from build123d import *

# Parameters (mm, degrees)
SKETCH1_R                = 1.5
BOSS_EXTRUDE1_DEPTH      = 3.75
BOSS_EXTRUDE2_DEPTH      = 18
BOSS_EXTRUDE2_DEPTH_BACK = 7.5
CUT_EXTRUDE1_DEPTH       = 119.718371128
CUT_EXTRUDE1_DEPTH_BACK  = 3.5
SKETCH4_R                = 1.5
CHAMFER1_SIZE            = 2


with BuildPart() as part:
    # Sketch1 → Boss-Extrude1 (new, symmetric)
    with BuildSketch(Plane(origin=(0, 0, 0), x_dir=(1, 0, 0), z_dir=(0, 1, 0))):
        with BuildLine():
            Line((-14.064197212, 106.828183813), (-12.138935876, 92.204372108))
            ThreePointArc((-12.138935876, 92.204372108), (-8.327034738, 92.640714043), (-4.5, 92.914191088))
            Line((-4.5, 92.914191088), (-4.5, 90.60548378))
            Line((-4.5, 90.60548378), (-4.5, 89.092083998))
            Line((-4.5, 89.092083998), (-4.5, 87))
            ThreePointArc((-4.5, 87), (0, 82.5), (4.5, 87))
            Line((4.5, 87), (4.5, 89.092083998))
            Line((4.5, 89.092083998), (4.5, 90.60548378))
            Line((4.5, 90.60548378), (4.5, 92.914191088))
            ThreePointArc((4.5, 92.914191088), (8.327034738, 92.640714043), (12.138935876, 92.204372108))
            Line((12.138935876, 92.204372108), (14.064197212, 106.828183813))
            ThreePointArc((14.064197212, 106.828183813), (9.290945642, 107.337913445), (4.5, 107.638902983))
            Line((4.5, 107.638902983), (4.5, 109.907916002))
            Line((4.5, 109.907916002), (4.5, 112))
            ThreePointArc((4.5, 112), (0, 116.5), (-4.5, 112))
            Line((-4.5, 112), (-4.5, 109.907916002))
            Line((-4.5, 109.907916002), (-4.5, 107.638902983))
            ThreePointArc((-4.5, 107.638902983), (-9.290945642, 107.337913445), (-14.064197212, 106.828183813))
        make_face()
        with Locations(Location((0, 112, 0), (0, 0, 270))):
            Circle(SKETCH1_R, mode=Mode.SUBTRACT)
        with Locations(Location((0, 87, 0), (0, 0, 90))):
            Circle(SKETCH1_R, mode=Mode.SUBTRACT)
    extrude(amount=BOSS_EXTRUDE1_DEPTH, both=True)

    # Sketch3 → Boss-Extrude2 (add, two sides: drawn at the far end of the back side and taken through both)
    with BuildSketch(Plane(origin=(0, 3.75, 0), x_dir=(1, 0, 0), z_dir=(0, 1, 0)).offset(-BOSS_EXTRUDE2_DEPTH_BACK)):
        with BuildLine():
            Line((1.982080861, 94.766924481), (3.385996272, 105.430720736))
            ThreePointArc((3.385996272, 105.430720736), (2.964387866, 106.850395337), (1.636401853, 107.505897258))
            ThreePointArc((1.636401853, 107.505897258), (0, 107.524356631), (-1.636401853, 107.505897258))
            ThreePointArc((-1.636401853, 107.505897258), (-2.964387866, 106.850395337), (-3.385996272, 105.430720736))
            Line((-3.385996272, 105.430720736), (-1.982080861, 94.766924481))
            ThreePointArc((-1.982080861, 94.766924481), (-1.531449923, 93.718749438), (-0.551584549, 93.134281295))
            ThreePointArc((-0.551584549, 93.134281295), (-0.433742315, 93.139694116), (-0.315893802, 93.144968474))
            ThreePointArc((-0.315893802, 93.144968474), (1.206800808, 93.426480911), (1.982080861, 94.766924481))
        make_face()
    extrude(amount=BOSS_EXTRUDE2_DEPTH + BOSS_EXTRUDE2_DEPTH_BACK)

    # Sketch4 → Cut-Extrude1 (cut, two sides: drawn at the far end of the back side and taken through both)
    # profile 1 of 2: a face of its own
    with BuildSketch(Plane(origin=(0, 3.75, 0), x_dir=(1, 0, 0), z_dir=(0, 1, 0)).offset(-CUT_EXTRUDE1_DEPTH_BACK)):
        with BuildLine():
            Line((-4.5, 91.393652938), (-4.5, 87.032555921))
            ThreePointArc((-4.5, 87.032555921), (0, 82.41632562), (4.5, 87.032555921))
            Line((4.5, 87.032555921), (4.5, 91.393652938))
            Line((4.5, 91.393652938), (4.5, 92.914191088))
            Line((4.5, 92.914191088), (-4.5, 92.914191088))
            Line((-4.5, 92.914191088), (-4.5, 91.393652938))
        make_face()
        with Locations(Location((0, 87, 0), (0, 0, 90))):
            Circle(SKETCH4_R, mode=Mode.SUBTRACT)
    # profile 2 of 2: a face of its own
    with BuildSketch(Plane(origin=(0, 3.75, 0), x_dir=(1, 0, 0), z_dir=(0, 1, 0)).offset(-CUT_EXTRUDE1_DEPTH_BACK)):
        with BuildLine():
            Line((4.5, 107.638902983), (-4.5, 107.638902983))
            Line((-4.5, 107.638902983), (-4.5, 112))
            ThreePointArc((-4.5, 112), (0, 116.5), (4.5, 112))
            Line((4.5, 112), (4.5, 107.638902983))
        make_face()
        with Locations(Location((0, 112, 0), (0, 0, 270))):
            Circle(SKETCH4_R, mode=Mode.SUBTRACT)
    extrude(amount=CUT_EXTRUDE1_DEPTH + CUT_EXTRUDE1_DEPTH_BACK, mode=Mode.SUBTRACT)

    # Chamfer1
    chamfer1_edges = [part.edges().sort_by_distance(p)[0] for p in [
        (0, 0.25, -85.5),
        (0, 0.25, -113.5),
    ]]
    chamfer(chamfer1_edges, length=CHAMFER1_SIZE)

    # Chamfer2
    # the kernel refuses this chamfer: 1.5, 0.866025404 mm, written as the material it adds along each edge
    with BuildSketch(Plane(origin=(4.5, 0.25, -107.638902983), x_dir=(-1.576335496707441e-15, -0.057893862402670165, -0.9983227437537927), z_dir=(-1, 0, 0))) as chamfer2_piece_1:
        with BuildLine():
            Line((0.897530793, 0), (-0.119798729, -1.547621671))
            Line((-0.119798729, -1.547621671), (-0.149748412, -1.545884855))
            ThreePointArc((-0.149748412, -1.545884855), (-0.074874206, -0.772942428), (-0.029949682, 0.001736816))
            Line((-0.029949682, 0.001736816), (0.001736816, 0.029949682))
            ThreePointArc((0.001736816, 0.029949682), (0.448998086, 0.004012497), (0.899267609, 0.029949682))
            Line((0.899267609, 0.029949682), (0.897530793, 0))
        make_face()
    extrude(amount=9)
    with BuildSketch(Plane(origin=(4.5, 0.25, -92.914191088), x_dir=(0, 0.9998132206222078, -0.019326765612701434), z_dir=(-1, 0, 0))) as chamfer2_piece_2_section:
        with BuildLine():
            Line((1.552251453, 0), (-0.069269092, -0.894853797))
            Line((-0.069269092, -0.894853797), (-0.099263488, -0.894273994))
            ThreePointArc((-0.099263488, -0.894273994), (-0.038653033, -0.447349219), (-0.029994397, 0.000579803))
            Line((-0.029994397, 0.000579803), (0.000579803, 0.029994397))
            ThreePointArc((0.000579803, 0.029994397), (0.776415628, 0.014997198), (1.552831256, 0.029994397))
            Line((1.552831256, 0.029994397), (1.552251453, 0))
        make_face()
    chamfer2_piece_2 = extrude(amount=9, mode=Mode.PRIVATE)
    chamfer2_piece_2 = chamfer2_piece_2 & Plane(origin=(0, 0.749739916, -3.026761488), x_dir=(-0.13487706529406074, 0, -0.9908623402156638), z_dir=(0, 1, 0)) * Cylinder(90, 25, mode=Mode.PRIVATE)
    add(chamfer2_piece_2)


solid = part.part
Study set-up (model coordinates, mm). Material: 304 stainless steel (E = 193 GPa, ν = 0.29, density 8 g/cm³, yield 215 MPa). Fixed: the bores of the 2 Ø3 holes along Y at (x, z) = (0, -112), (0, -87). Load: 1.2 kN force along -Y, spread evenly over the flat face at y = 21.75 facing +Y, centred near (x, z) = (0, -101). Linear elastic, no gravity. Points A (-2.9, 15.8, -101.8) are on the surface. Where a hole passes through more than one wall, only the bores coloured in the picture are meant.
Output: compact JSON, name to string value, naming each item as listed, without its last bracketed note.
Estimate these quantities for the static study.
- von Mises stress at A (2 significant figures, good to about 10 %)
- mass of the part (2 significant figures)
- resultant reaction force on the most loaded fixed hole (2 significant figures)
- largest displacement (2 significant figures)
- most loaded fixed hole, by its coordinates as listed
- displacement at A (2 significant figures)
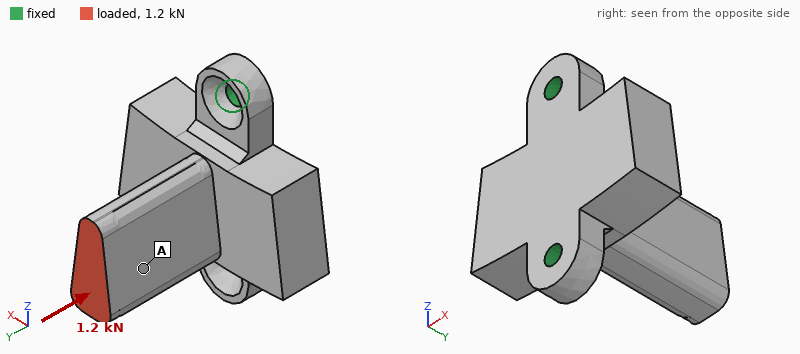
{"von Mises stress at A": "16 MPa", "mass of the part": "38 g", "resultant reaction force on the most loaded fixed hole": "820 N", "largest displacement": "5.4 µm", "most loaded fixed hole, by its coordinates as listed": "(0, -112)", "displacement at A": "4.6 µm"}
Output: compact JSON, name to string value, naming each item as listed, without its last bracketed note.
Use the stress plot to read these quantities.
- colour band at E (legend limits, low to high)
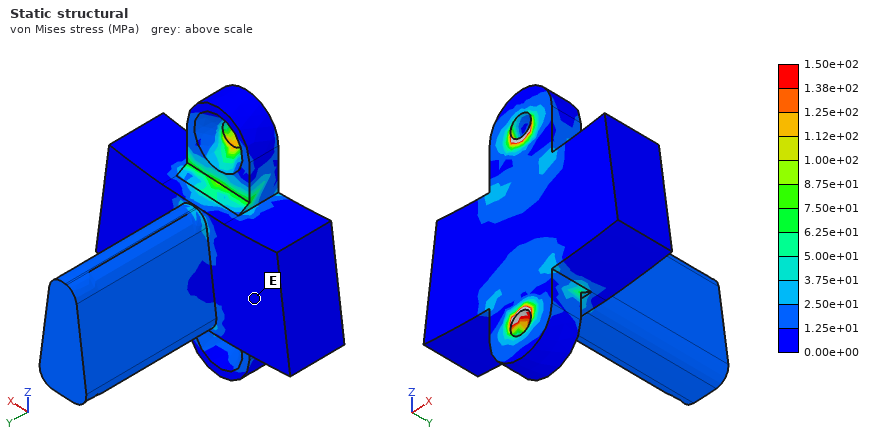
{"colour band at E": "0.00e+00 to 1.25e+01 MPa"}
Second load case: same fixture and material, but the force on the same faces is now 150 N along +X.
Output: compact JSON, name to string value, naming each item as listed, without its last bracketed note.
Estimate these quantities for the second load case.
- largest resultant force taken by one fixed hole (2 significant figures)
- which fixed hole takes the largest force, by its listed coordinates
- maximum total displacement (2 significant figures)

{"largest resultant force taken by one fixed hole": "86 N", "which fixed hole takes the largest force, by its listed coordinates": "(0, -112)", "maximum total displacement": "43 µm"}
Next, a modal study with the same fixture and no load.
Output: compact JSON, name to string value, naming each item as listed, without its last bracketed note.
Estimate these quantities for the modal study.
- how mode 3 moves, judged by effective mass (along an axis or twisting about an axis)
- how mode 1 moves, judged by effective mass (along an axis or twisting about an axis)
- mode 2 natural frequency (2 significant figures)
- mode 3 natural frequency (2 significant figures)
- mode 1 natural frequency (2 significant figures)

{"how mode 3 moves, judged by effective mass": "along Y", "how mode 1 moves, judged by effective mass": "along X", "mode 2 natural frequency": "13 kHz", "mode 3 natural frequency": "15 kHz", "mode 1 natural frequency": "3800 Hz"}
